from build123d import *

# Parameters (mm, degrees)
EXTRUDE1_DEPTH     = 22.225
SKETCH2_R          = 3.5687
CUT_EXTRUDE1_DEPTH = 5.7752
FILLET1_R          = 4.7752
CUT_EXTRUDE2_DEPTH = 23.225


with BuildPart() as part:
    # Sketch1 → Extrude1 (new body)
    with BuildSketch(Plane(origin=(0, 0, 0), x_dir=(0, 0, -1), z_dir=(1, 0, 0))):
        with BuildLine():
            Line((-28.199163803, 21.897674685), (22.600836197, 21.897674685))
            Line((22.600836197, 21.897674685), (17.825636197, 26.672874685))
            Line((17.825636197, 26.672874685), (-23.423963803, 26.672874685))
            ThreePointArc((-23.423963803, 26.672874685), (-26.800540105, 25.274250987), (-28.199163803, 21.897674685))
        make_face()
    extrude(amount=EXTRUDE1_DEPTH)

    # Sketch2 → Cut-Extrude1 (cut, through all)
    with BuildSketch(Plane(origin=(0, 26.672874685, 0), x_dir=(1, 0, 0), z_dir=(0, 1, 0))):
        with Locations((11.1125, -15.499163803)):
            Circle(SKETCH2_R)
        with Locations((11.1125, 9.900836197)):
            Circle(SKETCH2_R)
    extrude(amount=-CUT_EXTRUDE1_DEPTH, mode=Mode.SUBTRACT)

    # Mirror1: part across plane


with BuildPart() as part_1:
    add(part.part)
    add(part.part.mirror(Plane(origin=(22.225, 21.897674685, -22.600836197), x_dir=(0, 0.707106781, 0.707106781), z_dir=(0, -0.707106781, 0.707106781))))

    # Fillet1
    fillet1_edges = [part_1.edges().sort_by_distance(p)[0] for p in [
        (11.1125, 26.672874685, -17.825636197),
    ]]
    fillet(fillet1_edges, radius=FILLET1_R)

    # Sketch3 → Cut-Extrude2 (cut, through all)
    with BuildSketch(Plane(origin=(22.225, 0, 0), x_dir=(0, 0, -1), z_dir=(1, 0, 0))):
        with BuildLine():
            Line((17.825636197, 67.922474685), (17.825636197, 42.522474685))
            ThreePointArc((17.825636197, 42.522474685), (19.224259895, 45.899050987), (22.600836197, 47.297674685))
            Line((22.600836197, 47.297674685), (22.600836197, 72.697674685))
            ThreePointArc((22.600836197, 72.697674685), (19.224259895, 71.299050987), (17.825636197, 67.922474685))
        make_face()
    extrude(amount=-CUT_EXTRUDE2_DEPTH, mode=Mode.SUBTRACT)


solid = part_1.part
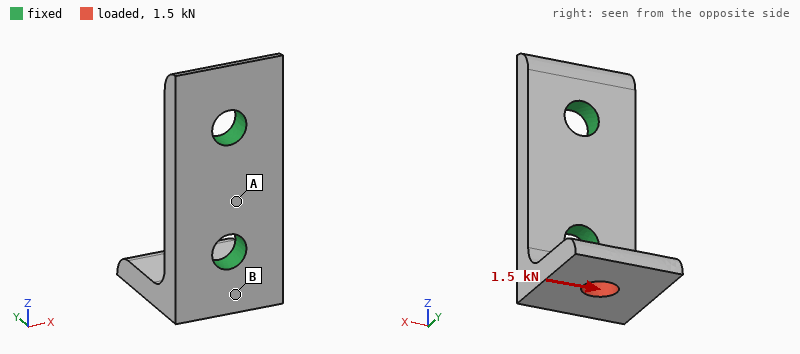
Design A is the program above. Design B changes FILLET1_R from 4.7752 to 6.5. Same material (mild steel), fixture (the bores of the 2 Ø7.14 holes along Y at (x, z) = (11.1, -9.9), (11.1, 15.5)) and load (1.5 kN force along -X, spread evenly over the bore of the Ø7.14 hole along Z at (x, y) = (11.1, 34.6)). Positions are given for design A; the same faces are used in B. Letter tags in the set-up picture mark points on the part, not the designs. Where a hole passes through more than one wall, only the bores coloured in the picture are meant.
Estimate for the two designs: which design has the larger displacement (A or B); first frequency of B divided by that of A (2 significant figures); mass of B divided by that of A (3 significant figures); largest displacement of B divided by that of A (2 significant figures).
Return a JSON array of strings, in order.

["A", "1.1", "1.01", "0.88"]
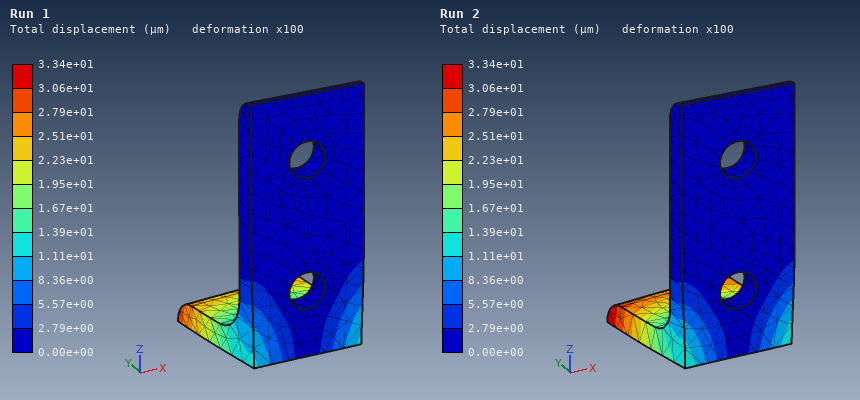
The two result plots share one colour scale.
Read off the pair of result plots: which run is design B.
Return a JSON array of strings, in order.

["Run 1"]
